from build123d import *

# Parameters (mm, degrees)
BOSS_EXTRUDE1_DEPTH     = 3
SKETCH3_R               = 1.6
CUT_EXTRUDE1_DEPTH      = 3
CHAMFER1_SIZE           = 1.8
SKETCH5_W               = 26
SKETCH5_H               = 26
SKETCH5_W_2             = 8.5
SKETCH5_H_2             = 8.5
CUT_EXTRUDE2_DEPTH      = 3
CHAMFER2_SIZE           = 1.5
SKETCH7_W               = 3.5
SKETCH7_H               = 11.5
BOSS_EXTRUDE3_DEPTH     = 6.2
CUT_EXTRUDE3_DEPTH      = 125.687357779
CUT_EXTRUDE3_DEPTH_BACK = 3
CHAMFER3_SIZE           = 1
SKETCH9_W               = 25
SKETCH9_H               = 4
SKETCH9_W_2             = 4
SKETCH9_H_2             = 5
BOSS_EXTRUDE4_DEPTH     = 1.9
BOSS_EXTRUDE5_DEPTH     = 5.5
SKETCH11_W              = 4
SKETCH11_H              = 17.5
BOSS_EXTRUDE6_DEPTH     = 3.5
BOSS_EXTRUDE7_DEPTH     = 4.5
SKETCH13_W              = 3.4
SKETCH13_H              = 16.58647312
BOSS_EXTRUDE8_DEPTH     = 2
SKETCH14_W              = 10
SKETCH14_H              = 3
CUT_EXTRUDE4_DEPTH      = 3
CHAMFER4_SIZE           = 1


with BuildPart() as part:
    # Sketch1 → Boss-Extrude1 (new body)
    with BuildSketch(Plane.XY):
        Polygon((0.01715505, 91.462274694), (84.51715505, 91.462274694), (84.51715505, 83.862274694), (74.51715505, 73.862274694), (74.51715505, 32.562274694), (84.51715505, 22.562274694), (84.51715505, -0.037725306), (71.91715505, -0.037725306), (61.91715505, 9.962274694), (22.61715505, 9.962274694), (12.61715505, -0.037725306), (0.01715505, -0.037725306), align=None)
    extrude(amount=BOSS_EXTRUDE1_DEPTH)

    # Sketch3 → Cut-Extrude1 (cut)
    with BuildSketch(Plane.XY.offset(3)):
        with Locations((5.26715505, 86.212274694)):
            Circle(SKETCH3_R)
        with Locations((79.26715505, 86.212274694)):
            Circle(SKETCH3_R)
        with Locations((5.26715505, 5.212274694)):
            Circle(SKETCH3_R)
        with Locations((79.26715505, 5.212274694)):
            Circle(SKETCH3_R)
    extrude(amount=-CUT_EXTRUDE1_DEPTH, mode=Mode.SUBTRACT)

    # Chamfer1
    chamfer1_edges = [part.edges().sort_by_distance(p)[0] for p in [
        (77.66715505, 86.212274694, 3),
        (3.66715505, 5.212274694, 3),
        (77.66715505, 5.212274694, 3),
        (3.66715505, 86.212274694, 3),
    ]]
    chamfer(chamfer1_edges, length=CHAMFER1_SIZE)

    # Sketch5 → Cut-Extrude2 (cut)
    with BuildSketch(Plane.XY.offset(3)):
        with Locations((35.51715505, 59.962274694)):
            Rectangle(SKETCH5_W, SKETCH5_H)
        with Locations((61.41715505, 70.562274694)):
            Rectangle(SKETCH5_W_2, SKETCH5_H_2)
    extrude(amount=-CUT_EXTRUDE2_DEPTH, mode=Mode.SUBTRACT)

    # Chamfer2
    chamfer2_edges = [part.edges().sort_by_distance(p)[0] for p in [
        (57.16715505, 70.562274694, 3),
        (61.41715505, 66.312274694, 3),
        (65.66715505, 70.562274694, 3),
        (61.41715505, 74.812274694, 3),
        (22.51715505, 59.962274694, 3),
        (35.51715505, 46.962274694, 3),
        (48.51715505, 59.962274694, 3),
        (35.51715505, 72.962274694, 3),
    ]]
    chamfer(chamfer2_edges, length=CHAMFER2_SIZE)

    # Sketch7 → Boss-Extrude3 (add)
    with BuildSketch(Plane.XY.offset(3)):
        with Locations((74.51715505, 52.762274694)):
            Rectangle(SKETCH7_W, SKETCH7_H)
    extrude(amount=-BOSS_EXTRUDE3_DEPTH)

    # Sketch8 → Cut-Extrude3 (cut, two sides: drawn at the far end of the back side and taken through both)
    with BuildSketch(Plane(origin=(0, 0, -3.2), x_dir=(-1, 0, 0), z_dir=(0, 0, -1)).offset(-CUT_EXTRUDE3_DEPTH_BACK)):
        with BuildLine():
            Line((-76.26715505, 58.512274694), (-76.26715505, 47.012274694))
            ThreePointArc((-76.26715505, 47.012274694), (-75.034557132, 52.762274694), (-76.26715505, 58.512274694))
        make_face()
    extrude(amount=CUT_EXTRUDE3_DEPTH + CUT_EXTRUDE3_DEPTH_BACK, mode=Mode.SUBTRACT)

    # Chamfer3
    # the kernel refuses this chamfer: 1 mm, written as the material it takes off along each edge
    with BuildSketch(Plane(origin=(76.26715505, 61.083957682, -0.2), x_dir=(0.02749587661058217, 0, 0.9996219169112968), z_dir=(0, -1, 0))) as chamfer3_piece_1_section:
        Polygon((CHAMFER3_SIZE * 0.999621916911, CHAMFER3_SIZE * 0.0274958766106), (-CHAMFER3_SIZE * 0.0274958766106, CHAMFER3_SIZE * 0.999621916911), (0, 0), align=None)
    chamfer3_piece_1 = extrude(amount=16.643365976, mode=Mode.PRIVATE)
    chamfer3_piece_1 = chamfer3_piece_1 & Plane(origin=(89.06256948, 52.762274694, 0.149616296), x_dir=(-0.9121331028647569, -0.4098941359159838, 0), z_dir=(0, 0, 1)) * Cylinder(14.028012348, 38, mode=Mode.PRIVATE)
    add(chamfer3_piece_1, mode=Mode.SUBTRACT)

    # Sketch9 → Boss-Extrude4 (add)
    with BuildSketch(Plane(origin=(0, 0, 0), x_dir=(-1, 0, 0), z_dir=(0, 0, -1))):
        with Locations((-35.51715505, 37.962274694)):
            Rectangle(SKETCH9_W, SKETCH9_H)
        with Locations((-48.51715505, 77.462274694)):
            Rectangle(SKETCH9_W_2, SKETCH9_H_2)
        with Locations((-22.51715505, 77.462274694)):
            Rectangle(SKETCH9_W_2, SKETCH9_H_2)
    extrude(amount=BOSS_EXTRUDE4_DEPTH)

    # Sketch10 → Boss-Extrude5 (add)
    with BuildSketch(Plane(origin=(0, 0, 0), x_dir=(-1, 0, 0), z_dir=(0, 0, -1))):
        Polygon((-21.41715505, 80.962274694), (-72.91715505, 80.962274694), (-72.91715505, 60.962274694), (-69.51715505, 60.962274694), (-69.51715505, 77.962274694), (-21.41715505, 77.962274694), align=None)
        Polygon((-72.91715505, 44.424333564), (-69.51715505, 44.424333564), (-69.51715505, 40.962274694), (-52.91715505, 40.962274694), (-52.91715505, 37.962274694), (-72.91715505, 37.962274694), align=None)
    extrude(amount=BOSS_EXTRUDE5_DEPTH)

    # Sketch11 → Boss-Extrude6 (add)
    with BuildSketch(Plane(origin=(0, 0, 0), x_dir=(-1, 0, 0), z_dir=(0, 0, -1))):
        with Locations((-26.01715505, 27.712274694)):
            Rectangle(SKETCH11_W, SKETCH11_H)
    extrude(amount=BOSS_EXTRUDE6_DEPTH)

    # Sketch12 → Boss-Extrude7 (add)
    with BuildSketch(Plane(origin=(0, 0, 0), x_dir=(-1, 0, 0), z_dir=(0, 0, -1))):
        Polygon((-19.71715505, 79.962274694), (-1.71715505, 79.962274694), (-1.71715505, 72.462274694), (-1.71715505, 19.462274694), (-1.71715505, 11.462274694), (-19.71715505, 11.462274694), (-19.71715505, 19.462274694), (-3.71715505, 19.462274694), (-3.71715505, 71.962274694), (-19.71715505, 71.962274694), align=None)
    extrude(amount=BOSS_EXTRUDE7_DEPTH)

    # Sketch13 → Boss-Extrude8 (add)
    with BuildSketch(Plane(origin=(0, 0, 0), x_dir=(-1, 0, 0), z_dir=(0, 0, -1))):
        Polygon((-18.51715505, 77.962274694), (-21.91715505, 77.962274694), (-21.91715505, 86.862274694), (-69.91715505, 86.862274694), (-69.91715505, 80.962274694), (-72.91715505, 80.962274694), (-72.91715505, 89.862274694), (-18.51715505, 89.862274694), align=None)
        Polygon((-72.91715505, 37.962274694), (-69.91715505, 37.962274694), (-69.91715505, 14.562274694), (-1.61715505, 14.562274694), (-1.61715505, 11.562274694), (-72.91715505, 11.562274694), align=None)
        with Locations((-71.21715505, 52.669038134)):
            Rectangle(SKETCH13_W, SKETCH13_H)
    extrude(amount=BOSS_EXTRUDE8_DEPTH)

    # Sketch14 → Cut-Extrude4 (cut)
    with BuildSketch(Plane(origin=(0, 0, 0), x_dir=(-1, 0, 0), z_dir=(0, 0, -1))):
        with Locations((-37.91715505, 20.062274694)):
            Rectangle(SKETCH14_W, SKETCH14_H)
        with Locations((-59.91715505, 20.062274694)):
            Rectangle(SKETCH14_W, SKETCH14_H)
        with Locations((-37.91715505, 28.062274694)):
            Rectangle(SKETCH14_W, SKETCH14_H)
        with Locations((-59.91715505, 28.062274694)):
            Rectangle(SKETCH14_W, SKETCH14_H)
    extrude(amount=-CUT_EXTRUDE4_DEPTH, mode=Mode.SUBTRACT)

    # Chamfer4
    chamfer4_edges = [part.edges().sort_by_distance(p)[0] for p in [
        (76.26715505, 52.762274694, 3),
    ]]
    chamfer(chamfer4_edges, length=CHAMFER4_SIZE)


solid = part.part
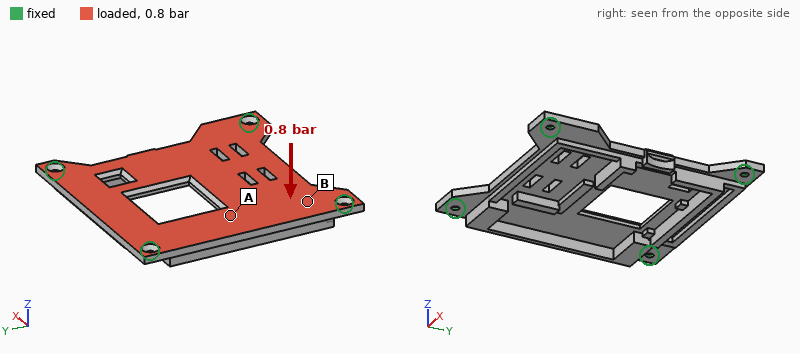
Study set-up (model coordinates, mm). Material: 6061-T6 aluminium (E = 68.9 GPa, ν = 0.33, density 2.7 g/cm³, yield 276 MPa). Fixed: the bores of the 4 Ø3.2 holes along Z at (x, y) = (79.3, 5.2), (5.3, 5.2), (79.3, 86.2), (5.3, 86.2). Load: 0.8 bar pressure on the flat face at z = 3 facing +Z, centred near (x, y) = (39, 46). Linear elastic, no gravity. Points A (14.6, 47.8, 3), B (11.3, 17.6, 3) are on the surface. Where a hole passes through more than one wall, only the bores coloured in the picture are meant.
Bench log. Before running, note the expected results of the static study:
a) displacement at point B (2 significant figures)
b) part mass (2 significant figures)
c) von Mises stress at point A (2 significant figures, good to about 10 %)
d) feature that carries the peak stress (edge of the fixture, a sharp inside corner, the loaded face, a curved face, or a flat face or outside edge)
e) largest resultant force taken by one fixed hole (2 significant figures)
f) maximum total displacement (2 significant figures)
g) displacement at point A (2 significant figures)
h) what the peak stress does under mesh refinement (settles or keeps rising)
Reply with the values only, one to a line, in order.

0.038 mm
60 g
17 MPa
edge of the fixture
130 N
0.13 mm
0.084 mm
keeps rising
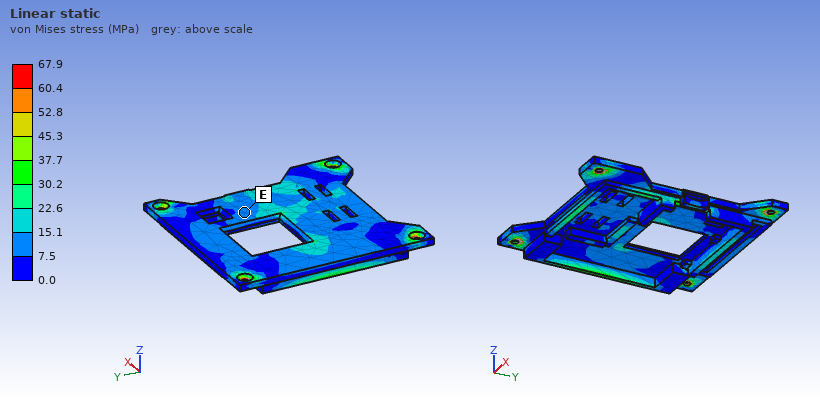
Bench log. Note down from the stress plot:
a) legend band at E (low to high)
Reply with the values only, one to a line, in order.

7.5 to 15.1 MPa
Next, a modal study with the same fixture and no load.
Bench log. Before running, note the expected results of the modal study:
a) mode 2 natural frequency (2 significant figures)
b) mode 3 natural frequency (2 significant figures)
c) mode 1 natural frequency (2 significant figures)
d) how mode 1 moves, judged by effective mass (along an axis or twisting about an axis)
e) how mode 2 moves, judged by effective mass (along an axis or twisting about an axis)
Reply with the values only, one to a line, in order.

2800 Hz
3300 Hz
1600 Hz
along Z
twisting about Y
